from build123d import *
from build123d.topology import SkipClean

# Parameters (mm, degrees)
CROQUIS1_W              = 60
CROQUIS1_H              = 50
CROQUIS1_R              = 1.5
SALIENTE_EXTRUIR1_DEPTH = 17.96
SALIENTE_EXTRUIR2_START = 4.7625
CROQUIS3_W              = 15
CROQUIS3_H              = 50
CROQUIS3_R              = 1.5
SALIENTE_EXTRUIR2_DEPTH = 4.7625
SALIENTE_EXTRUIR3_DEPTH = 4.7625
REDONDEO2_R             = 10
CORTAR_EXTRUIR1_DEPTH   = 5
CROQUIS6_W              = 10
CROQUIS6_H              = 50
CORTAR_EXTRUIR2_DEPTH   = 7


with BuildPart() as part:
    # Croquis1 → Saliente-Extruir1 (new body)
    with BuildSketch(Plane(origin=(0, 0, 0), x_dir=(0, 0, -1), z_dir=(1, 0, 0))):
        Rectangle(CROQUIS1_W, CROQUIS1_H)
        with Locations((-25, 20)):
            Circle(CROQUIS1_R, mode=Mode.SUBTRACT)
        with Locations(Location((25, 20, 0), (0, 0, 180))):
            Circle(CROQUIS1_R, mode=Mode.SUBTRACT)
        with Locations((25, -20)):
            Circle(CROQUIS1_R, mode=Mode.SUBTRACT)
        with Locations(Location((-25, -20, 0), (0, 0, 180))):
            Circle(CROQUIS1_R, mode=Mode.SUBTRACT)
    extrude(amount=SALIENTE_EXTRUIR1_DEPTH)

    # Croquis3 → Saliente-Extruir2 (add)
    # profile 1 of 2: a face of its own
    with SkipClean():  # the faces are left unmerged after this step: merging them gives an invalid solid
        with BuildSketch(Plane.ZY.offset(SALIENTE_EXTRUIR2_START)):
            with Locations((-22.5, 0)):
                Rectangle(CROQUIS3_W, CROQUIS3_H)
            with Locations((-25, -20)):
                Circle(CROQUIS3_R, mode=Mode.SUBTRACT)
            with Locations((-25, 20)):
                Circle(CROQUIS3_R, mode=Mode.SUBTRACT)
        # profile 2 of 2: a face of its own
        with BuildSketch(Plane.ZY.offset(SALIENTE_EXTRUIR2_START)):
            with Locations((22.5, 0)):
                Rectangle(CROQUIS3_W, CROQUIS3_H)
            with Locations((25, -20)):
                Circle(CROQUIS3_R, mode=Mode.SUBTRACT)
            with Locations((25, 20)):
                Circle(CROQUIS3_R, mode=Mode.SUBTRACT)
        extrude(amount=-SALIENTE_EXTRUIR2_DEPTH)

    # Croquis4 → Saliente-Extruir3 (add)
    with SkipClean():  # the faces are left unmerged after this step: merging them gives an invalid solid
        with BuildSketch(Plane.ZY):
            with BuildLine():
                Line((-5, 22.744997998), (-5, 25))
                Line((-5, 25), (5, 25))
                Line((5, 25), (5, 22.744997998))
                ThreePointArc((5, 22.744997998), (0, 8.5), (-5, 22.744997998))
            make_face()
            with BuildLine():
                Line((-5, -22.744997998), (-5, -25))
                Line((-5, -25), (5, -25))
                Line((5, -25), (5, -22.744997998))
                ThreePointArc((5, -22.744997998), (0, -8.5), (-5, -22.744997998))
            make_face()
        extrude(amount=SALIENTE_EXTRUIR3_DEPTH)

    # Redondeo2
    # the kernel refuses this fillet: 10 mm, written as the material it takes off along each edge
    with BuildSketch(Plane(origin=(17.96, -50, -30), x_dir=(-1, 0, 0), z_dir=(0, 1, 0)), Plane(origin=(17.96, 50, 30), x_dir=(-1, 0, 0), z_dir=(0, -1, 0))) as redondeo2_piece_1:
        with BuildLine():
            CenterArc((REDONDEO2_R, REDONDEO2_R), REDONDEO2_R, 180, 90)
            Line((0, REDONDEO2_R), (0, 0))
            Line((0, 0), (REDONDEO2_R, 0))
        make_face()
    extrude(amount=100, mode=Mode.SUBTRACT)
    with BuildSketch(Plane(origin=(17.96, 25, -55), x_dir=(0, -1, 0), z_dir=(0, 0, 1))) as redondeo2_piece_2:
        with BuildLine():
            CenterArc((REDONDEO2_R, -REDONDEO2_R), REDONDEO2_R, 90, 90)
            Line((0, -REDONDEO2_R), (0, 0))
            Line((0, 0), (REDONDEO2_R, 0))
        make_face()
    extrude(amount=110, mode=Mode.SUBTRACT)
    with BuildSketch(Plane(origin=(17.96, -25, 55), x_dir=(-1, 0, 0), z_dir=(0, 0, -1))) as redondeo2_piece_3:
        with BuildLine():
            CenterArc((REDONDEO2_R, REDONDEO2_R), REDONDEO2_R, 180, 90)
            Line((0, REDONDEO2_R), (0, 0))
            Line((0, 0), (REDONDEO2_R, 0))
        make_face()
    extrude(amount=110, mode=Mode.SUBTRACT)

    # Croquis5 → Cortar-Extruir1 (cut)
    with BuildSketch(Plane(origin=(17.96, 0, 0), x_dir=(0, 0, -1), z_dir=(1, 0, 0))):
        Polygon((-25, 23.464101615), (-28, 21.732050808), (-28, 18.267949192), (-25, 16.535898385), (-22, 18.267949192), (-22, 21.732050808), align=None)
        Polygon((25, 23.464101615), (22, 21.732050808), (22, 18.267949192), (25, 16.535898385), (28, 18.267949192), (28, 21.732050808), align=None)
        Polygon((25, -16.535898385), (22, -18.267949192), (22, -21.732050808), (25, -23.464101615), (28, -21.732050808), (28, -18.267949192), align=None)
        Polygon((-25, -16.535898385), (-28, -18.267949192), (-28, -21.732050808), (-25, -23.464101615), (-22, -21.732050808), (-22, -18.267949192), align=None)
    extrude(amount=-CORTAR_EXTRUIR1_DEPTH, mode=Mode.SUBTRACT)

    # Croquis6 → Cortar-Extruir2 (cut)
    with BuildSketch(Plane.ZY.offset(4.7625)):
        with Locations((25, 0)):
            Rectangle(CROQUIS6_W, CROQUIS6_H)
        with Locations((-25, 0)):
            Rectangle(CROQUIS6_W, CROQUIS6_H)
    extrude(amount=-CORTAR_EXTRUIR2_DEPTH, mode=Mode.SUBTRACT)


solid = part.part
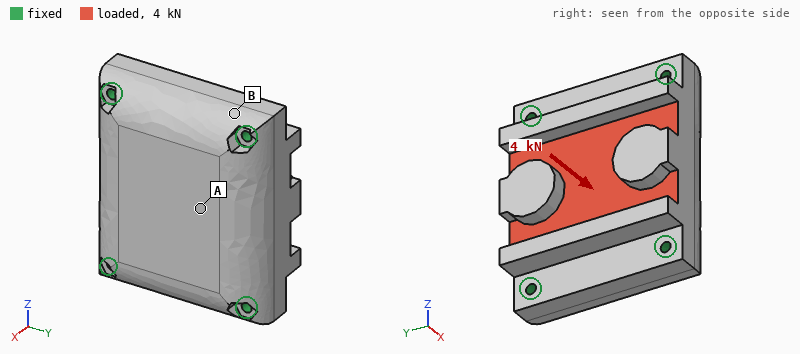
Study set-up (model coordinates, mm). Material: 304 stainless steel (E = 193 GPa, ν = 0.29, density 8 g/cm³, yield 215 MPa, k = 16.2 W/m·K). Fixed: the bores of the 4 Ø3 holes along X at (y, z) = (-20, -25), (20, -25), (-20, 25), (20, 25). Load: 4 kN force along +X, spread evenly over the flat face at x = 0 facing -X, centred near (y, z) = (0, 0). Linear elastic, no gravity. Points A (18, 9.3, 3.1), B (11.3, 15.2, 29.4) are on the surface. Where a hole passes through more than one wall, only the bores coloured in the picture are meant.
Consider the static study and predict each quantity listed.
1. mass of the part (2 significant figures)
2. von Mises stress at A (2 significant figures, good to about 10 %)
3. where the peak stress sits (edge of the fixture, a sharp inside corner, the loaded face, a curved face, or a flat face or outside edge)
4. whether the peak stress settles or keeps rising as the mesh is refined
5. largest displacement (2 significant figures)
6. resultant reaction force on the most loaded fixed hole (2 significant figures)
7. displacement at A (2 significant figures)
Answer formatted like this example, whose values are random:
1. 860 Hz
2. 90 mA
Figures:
1. 410 g
2. 8.4 MPa
3. edge of the fixture
4. keeps rising
5. 2.4 µm
6. 1.0 kN
7. 2.1 µm
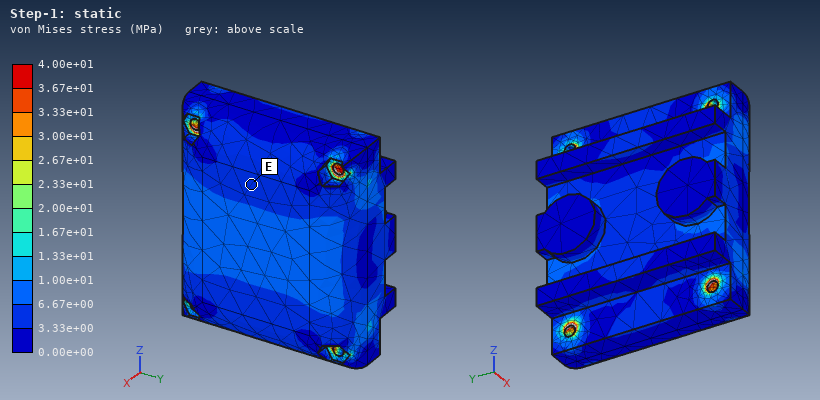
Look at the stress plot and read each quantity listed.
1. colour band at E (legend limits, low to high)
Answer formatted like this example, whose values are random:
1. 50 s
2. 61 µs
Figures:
1. 3.33e+00 to 6.67e+00 MPa
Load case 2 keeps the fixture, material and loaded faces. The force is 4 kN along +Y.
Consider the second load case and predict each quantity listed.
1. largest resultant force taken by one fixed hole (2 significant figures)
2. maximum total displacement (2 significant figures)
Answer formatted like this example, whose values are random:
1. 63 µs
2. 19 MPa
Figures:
1. 1.2 kN
2. 2.0 µm
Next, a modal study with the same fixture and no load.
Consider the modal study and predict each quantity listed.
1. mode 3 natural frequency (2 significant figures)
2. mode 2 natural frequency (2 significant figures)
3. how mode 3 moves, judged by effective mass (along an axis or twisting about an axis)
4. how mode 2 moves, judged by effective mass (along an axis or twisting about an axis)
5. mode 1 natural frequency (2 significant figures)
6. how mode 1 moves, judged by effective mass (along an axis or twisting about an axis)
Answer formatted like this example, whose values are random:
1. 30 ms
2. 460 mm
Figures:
1. 21 kHz
2. 18 kHz
3. along Y
4. along Y
5. 13 kHz
6. along X
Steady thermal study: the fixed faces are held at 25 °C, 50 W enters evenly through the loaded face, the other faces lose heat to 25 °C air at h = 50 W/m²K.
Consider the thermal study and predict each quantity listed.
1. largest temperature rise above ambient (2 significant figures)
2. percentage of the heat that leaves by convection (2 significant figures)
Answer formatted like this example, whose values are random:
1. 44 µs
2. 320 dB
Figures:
1. 61 K
2. 26 %
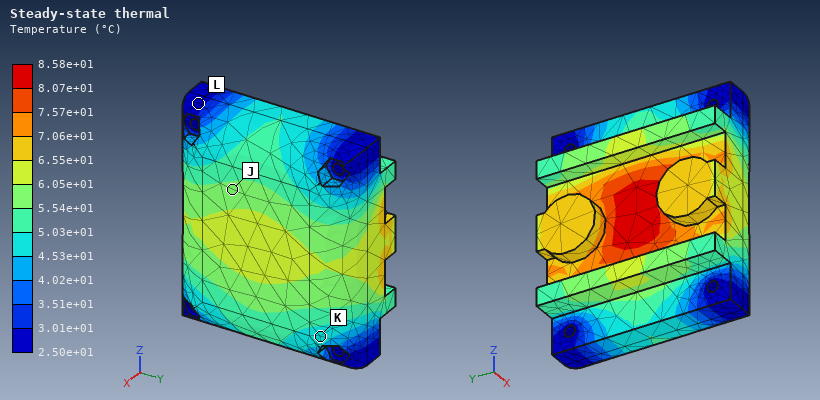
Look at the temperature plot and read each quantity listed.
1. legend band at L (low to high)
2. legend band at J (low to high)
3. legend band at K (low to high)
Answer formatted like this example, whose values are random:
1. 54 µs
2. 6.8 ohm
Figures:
1. 2.50e+01 to 3.01e+01 °C
2. 5.54e+01 to 6.05e+01 °C
3. 4.53e+01 to 5.03e+01 °C
